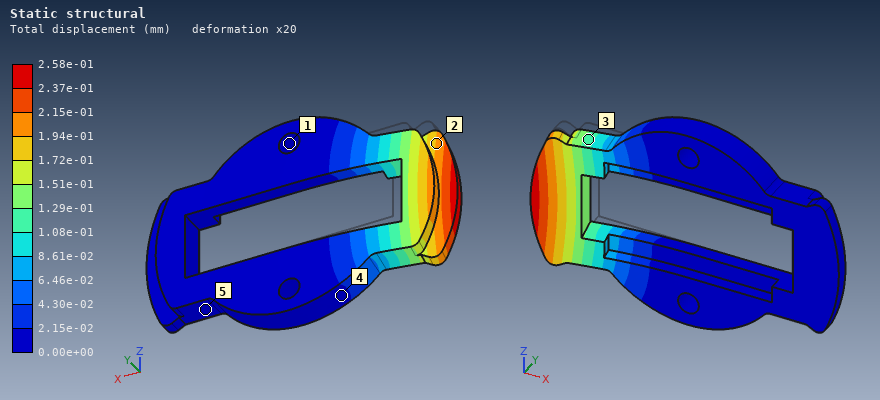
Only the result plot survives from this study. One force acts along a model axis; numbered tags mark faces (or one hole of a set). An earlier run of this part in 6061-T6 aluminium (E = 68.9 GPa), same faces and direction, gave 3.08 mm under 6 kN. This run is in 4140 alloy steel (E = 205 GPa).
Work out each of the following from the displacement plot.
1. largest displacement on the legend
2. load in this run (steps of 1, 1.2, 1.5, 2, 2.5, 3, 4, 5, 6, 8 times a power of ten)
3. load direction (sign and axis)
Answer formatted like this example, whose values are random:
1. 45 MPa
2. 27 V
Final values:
1. 2.58e-01 mm
2. 1.5 kN
3. -Y
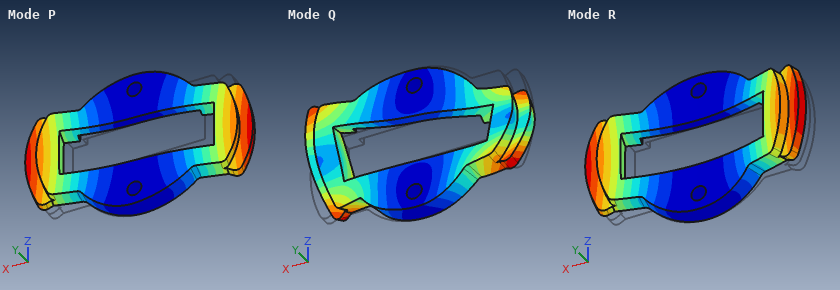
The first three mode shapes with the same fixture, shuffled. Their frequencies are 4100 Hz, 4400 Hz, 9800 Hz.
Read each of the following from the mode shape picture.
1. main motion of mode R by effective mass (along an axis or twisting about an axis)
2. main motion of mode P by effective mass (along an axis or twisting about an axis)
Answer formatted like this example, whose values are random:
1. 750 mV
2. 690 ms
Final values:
1. along Y
2. twisting about Z
